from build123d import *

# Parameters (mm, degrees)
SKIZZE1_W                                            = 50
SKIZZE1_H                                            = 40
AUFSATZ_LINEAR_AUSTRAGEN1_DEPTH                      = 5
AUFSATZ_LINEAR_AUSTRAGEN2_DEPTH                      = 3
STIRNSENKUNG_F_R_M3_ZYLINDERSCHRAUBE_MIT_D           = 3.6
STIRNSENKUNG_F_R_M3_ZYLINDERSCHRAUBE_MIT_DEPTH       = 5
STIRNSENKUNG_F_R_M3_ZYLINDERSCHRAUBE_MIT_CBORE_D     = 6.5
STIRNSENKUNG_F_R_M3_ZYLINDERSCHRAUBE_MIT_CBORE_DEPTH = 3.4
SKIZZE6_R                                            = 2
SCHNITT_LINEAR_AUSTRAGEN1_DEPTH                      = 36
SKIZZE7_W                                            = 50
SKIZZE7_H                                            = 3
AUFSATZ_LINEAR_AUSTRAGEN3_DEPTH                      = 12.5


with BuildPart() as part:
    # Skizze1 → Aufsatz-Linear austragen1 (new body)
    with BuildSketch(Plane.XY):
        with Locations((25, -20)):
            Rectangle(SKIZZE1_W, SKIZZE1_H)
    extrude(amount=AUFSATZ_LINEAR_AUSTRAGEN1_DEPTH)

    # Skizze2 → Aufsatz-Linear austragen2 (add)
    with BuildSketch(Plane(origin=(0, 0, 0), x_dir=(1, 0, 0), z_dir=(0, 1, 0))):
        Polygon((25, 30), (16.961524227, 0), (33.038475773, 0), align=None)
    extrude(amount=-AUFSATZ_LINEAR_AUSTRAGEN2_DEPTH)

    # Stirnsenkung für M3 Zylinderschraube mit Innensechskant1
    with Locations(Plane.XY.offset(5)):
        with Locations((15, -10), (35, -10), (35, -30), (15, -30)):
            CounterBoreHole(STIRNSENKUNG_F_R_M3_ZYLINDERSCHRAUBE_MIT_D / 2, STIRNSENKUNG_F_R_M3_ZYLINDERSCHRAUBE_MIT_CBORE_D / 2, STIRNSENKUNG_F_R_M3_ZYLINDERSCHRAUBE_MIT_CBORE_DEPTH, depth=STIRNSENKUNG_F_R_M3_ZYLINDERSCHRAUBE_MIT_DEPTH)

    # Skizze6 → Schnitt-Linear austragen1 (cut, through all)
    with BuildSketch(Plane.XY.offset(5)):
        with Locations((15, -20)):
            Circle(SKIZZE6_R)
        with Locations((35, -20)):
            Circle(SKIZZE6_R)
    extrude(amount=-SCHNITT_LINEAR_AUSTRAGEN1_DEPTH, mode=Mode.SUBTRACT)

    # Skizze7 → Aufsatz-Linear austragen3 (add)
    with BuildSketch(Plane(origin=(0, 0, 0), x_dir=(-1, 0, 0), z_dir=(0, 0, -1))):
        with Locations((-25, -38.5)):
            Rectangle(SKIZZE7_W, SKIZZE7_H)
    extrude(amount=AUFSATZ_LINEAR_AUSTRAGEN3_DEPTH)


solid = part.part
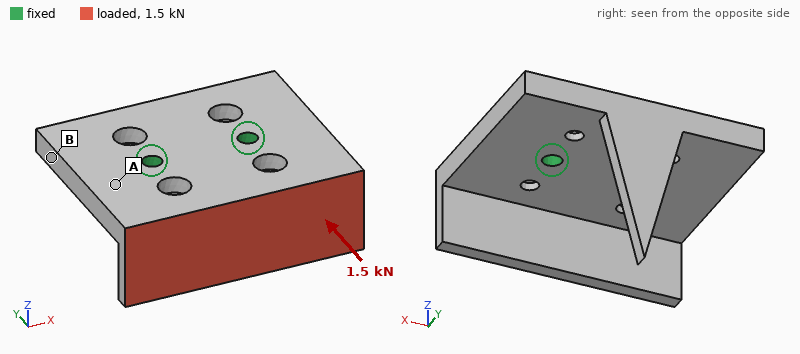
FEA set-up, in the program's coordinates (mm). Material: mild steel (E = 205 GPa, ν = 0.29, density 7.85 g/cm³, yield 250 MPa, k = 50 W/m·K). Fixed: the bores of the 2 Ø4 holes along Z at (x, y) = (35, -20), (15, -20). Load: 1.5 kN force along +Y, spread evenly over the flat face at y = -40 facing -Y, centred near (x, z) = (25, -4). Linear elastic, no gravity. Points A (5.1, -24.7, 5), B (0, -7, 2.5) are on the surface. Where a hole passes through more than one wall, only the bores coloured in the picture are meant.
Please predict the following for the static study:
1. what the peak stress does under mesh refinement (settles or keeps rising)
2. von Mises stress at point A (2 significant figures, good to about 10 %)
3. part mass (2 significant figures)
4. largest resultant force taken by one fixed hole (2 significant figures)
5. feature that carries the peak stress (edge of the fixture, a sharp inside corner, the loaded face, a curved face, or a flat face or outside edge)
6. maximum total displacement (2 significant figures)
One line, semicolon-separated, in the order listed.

keeps rising; 35 MPa; 94 g; 750 N; edge of the fixture; 50 µm
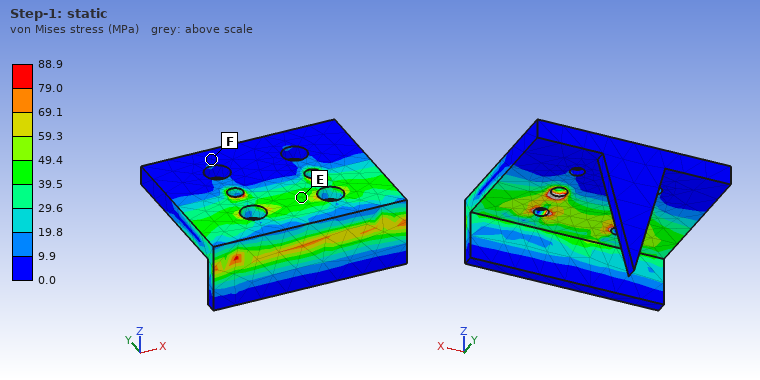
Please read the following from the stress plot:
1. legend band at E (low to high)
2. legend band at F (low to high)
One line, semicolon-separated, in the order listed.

39.5 to 49.4 MPa; 0.0 to 9.9 MPa
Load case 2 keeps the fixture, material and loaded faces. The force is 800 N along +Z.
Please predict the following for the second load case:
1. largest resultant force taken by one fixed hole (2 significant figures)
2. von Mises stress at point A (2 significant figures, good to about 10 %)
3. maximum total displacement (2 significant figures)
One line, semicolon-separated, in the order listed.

400 N; 46 MPa; 41 µm
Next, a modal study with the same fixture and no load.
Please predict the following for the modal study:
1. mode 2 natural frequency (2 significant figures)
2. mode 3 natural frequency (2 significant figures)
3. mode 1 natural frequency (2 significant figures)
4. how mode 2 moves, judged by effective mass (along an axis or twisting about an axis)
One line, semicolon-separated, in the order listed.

5100 Hz; 6500 Hz; 4300 Hz; along Z
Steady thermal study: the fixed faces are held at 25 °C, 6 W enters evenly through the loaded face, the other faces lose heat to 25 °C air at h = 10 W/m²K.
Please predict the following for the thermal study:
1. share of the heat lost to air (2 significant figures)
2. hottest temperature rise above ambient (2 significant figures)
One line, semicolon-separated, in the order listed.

5.1 %; 15 K
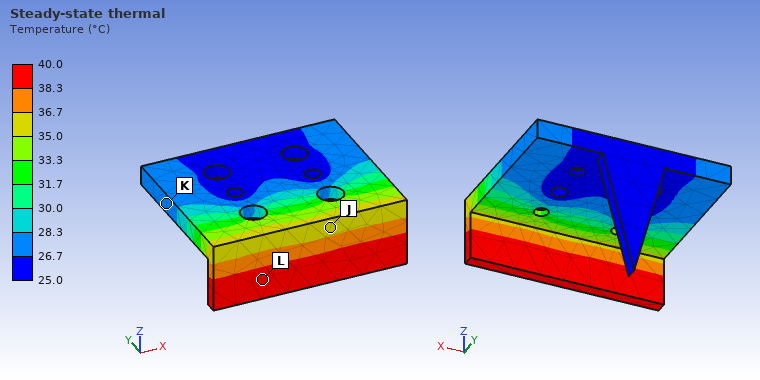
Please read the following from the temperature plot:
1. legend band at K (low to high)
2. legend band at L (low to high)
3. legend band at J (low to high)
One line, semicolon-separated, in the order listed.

26.7 to 28.3 °C; 38.3 to 40.0 °C; 35.0 to 36.7 °C
